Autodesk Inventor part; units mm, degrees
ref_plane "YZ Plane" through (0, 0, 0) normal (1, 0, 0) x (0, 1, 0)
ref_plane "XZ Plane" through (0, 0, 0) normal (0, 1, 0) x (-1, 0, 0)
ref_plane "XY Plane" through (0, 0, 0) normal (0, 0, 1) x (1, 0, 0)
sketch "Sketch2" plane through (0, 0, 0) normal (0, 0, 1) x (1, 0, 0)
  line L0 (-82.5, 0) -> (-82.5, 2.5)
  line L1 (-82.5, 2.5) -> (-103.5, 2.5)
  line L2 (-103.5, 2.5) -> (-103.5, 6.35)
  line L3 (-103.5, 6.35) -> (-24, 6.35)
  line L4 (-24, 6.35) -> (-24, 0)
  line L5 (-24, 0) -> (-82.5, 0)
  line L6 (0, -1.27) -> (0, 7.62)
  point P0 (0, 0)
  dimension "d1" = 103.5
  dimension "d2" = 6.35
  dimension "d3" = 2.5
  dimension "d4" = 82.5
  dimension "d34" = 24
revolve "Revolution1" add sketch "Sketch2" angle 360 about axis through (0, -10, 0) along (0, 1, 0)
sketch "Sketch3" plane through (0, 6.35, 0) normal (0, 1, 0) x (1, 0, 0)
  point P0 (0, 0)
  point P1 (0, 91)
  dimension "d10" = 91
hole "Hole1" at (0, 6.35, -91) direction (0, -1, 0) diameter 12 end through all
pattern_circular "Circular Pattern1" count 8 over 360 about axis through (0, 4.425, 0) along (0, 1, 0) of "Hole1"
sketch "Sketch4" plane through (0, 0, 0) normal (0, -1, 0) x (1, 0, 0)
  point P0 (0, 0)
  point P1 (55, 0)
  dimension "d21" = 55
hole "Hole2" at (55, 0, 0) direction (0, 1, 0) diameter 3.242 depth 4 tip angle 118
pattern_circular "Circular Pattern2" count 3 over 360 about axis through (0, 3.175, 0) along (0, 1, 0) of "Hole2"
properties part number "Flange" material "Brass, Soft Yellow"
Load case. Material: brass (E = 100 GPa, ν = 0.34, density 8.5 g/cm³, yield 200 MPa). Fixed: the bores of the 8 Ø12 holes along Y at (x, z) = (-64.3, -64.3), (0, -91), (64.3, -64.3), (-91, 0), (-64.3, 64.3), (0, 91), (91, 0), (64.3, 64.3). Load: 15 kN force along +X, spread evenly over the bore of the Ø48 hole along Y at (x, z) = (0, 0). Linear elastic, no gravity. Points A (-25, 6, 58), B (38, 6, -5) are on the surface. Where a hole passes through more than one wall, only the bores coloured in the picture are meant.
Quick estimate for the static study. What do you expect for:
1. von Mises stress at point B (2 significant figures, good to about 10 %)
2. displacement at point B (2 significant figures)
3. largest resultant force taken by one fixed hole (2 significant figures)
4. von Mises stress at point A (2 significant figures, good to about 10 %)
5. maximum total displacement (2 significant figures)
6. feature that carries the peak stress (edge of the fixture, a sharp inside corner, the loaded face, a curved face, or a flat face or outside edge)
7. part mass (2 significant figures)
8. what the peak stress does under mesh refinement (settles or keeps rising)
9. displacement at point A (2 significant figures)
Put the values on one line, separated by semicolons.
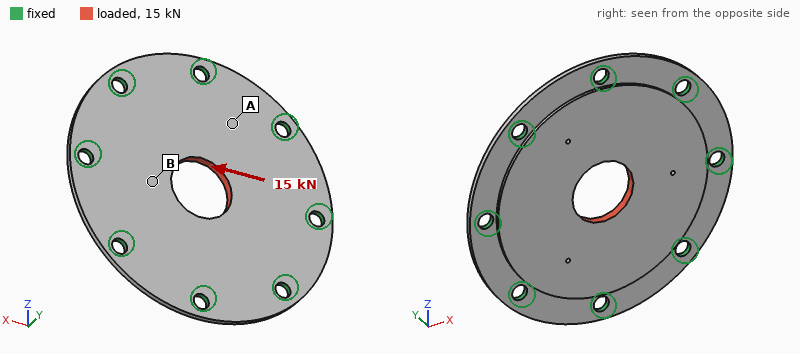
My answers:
15 MPa; 11 µm; 3.0 kN; 7.2 MPa; 13 µm; edge of the fixture; 1.4 kg; keeps rising; 4.3 µm
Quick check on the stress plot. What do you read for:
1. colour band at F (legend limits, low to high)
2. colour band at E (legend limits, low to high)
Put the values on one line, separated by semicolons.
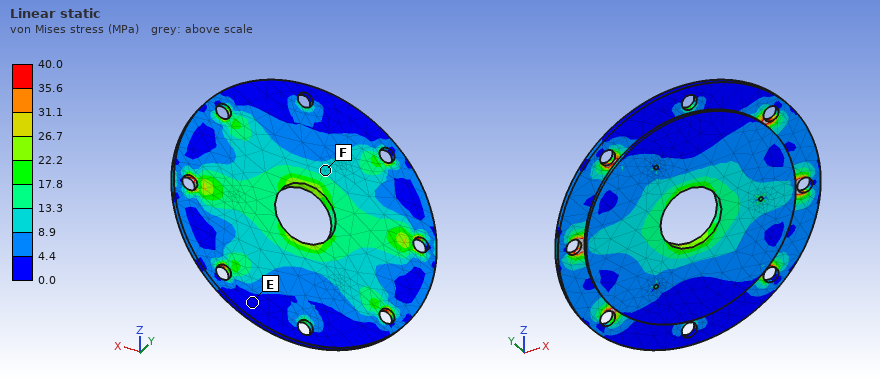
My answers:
8.9 to 13.3 MPa; 0.0 to 4.4 MPa
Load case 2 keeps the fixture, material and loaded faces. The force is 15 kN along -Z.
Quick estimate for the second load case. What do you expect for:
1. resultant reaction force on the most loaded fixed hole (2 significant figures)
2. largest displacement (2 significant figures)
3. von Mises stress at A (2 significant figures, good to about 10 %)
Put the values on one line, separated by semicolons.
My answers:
3.0 kN; 13 µm; 8.9 MPa
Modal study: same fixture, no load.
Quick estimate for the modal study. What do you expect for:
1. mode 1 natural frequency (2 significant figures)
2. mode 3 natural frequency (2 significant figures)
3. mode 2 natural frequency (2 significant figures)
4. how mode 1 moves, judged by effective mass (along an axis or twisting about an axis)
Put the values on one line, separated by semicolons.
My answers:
1000 Hz; 2000 Hz; 2000 Hz; along Y
